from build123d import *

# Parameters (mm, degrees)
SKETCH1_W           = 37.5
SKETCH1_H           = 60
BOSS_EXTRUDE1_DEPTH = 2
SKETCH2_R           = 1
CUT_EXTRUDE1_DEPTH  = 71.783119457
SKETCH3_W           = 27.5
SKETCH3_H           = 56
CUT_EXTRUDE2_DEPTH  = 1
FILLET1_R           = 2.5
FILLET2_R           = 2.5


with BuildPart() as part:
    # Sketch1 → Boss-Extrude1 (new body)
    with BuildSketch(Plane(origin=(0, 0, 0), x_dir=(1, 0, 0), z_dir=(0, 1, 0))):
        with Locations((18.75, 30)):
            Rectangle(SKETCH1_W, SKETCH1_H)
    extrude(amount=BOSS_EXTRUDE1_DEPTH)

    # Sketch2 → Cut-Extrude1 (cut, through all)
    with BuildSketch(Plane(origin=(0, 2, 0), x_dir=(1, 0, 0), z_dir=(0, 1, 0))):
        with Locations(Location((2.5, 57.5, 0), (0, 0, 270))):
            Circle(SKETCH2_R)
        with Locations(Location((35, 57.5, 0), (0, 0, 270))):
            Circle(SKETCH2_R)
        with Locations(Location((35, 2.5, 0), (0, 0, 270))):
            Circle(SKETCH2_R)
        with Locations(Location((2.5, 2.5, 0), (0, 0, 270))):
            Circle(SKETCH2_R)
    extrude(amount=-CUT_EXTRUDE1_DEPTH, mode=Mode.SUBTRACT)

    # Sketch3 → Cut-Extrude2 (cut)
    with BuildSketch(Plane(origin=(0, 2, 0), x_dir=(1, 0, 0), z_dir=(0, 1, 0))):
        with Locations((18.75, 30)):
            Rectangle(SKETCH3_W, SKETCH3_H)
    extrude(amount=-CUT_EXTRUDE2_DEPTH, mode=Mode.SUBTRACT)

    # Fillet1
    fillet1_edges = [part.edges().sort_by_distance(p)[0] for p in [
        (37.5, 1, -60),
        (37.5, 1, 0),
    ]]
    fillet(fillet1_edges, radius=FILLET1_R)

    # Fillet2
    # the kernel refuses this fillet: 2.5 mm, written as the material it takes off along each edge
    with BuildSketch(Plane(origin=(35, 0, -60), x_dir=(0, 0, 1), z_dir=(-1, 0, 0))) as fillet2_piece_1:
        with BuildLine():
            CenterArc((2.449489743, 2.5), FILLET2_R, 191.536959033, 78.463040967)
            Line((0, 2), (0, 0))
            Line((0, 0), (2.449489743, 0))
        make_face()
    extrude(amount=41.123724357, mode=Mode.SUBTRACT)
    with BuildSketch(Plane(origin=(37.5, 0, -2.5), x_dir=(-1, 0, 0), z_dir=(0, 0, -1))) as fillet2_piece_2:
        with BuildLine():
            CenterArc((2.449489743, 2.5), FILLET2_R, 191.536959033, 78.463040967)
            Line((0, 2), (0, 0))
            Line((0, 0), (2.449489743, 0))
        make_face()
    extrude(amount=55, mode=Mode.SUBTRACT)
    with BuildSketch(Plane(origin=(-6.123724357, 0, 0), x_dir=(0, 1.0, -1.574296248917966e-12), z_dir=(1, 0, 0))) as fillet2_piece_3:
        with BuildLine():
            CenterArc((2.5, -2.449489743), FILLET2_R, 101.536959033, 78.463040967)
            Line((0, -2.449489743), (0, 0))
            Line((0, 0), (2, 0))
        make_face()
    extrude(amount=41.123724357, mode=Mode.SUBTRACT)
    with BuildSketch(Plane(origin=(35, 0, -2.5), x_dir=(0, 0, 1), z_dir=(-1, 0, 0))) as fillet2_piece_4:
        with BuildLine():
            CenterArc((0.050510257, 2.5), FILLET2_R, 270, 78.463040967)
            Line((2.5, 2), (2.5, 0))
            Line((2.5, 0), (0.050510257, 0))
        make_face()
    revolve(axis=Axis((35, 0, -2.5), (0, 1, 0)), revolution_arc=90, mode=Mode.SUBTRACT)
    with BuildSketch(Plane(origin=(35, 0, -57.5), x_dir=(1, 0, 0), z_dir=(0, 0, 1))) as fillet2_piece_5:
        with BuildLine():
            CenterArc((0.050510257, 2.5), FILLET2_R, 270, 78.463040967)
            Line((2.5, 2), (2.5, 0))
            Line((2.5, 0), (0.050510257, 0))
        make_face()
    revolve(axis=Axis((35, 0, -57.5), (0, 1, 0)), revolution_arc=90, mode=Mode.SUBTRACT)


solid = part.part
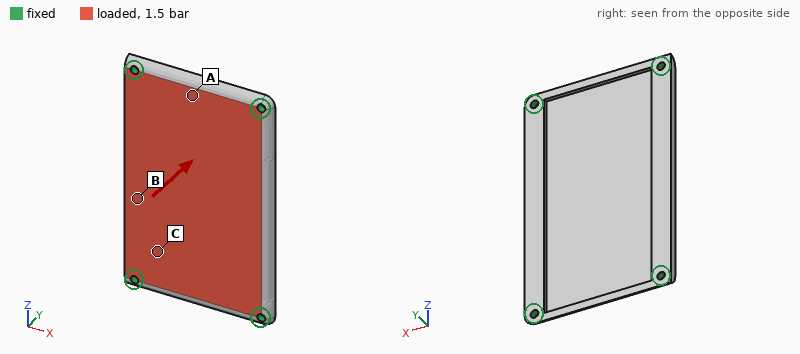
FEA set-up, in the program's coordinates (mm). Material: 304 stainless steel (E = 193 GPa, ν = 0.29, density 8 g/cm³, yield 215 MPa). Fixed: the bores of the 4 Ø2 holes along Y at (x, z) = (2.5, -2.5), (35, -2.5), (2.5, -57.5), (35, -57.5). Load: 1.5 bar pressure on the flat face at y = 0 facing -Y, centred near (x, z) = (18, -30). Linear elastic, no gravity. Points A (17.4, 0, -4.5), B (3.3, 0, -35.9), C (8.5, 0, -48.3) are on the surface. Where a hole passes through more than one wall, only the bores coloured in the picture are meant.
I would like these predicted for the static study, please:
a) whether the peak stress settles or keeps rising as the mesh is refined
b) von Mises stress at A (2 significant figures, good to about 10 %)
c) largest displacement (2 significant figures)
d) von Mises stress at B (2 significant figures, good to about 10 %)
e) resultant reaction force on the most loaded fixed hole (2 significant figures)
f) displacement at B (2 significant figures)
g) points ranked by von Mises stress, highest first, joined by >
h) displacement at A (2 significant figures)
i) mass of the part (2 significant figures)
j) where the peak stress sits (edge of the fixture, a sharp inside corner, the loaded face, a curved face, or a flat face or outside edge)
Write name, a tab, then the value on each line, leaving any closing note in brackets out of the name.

whether the peak stress settles or keeps rising as the mesh is refined	keeps rising
von Mises stress at A	23 MPa
largest displacement	99 µm
von Mises stress at B	51 MPa
resultant reaction force on the most loaded fixed hole	140 N
displacement at B	62 µm
points ranked by von Mises stress, highest first, joined by >	B > A > C
displacement at A	17 µm
mass of the part	22 g
where the peak stress sits	edge of the fixture
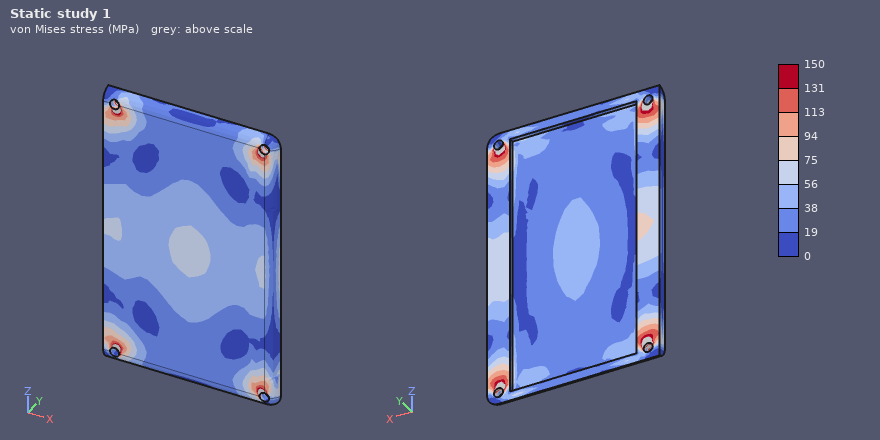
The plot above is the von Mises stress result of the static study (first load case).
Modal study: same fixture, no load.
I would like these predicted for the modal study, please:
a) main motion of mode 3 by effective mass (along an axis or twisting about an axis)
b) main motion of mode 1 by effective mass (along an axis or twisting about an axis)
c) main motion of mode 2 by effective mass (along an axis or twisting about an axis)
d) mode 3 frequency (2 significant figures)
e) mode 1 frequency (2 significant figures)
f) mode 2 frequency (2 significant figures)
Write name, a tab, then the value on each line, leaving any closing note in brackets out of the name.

main motion of mode 3 by effective mass	twisting about X
main motion of mode 1 by effective mass	along Y
main motion of mode 2 by effective mass	twisting about Z
mode 3 frequency	5600 Hz
mode 1 frequency	2500 Hz
mode 2 frequency	3600 Hz
